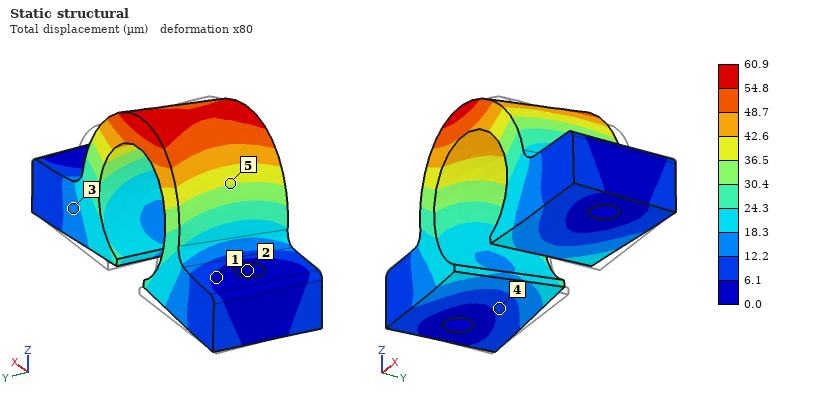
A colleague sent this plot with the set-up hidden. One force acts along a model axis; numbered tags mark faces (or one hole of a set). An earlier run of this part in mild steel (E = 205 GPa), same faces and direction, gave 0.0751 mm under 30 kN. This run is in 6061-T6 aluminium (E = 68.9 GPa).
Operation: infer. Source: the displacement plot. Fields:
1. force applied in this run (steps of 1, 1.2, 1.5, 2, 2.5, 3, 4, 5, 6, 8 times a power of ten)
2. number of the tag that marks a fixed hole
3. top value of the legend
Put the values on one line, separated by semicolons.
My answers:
8 kN; 2; 60.9 µm
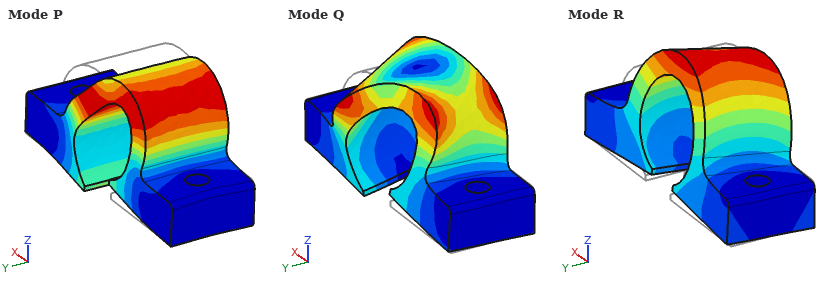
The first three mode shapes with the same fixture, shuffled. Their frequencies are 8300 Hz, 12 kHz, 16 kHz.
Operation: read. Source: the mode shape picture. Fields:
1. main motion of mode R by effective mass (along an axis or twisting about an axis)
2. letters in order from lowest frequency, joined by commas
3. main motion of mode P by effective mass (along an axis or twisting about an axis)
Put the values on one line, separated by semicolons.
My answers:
along Y; R, P, Q; along X
